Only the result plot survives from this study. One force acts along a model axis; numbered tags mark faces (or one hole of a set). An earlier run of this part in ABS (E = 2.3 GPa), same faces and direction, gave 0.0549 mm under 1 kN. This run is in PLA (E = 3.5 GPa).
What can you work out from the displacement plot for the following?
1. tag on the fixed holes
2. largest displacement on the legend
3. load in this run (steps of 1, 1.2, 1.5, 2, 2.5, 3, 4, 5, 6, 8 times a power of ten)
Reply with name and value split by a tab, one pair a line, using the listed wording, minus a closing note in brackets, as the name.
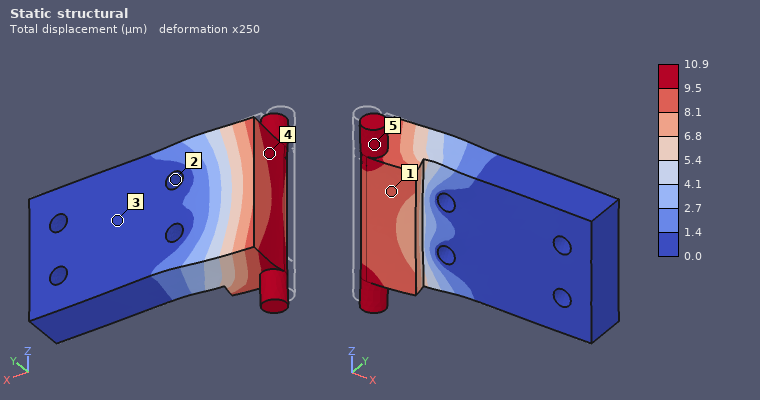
tag on the fixed holes	2
largest displacement on the legend	10.9 µm
load in this run	300 N
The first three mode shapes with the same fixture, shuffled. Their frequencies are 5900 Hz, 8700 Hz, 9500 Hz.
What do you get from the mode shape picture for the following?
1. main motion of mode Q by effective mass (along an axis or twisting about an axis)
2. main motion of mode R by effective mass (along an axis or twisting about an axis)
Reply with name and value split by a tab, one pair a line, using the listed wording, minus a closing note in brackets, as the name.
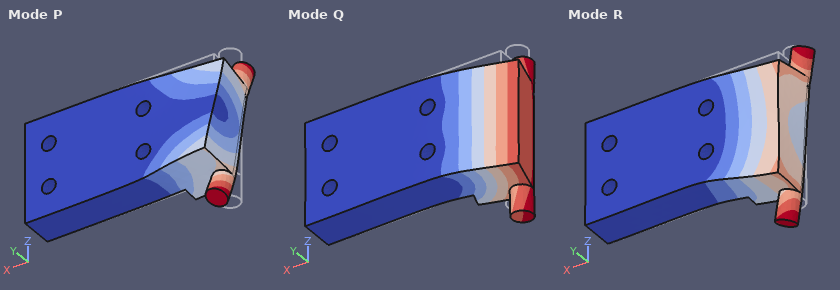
main motion of mode Q by effective mass	along Y
main motion of mode R by effective mass	along Z
